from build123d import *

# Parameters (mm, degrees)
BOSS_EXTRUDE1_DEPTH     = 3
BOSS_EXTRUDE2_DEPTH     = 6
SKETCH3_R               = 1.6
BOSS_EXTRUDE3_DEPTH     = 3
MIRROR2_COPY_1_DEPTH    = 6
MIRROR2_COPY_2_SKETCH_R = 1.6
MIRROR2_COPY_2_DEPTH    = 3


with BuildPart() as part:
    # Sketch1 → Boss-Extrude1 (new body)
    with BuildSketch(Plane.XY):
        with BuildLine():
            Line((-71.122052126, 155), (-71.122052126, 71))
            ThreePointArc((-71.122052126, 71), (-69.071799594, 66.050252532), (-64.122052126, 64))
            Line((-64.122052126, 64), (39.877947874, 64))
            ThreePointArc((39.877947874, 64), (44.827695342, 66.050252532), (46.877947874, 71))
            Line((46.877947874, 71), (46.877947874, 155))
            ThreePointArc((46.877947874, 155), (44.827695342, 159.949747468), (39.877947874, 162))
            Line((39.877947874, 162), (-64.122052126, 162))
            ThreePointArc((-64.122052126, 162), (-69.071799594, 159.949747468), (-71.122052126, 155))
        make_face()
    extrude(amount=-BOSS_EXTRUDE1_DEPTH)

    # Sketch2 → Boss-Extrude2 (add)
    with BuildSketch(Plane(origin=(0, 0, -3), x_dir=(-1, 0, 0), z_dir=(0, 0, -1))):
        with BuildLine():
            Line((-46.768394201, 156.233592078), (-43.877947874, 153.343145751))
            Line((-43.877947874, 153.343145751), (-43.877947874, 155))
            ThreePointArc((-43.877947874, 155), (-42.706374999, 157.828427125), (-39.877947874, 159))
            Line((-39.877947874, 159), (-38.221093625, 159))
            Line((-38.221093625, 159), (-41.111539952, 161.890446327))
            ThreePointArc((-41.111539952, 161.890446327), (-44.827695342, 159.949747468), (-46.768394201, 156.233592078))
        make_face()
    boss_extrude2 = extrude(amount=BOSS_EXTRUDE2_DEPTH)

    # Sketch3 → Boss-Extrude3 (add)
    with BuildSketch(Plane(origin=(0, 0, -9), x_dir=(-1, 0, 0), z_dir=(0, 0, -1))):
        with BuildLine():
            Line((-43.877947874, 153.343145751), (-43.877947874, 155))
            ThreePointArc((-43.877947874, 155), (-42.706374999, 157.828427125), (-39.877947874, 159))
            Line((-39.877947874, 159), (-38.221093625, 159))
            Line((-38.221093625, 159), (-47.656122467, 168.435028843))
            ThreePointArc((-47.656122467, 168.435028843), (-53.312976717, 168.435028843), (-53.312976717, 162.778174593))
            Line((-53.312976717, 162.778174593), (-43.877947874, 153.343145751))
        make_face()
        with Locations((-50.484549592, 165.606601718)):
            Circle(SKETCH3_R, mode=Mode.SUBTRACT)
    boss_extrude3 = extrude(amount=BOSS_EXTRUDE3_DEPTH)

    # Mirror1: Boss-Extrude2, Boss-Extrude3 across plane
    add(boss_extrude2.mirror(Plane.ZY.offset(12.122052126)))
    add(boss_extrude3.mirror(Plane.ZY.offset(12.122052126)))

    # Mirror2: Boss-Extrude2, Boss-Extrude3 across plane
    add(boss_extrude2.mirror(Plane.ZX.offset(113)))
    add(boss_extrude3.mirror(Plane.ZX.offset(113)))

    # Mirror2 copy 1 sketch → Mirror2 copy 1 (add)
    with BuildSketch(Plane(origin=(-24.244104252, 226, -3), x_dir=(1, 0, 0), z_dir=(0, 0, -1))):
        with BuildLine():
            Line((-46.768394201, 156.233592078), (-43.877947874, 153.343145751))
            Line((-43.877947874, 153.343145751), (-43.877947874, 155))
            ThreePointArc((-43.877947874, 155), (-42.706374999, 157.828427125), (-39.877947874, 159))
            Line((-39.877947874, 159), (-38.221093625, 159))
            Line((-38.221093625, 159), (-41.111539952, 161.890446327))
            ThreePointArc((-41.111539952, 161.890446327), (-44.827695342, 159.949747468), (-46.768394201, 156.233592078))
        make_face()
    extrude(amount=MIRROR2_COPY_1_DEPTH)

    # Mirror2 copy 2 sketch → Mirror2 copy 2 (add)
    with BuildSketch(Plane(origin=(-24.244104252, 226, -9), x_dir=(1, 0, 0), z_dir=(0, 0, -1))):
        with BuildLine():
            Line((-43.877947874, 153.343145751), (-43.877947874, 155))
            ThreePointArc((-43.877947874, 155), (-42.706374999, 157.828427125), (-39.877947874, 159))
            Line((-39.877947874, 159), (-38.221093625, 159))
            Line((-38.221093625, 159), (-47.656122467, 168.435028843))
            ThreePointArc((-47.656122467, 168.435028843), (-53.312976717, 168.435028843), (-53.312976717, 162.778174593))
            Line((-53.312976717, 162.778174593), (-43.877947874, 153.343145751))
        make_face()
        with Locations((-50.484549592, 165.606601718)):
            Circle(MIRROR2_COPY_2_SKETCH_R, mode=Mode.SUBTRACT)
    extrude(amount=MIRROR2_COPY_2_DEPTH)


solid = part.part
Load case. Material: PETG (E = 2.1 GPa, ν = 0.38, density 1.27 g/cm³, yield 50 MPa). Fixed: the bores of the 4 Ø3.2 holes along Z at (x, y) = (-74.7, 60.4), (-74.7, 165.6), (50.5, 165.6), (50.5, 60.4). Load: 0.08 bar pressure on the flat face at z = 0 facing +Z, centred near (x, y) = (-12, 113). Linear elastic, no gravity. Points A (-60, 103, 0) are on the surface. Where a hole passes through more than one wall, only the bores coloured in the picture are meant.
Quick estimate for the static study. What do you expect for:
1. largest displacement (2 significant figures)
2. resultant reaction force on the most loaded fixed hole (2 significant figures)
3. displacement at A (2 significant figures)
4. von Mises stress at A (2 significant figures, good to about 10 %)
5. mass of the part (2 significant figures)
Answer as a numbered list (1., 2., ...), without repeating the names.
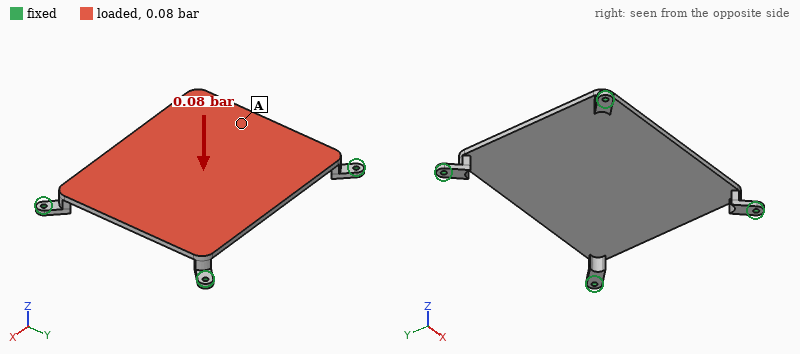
1. 1.7 mm
2. 54 N
3. 0.85 mm
4. 3.1 MPa
5. 46 g
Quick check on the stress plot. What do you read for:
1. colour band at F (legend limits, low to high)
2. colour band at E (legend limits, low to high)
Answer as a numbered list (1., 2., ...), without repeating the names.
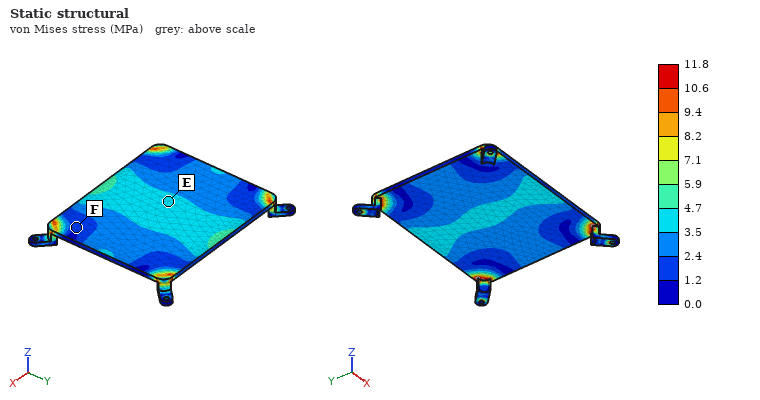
1. 1.2 to 2.4 MPa
2. 3.5 to 4.7 MPa
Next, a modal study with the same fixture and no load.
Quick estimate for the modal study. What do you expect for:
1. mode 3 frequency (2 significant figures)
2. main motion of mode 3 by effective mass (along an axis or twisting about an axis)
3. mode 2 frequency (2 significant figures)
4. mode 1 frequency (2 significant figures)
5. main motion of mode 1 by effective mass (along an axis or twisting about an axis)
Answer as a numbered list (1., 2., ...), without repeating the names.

1. 370 Hz
2. along X
3. 340 Hz
4. 200 Hz
5. along Z
